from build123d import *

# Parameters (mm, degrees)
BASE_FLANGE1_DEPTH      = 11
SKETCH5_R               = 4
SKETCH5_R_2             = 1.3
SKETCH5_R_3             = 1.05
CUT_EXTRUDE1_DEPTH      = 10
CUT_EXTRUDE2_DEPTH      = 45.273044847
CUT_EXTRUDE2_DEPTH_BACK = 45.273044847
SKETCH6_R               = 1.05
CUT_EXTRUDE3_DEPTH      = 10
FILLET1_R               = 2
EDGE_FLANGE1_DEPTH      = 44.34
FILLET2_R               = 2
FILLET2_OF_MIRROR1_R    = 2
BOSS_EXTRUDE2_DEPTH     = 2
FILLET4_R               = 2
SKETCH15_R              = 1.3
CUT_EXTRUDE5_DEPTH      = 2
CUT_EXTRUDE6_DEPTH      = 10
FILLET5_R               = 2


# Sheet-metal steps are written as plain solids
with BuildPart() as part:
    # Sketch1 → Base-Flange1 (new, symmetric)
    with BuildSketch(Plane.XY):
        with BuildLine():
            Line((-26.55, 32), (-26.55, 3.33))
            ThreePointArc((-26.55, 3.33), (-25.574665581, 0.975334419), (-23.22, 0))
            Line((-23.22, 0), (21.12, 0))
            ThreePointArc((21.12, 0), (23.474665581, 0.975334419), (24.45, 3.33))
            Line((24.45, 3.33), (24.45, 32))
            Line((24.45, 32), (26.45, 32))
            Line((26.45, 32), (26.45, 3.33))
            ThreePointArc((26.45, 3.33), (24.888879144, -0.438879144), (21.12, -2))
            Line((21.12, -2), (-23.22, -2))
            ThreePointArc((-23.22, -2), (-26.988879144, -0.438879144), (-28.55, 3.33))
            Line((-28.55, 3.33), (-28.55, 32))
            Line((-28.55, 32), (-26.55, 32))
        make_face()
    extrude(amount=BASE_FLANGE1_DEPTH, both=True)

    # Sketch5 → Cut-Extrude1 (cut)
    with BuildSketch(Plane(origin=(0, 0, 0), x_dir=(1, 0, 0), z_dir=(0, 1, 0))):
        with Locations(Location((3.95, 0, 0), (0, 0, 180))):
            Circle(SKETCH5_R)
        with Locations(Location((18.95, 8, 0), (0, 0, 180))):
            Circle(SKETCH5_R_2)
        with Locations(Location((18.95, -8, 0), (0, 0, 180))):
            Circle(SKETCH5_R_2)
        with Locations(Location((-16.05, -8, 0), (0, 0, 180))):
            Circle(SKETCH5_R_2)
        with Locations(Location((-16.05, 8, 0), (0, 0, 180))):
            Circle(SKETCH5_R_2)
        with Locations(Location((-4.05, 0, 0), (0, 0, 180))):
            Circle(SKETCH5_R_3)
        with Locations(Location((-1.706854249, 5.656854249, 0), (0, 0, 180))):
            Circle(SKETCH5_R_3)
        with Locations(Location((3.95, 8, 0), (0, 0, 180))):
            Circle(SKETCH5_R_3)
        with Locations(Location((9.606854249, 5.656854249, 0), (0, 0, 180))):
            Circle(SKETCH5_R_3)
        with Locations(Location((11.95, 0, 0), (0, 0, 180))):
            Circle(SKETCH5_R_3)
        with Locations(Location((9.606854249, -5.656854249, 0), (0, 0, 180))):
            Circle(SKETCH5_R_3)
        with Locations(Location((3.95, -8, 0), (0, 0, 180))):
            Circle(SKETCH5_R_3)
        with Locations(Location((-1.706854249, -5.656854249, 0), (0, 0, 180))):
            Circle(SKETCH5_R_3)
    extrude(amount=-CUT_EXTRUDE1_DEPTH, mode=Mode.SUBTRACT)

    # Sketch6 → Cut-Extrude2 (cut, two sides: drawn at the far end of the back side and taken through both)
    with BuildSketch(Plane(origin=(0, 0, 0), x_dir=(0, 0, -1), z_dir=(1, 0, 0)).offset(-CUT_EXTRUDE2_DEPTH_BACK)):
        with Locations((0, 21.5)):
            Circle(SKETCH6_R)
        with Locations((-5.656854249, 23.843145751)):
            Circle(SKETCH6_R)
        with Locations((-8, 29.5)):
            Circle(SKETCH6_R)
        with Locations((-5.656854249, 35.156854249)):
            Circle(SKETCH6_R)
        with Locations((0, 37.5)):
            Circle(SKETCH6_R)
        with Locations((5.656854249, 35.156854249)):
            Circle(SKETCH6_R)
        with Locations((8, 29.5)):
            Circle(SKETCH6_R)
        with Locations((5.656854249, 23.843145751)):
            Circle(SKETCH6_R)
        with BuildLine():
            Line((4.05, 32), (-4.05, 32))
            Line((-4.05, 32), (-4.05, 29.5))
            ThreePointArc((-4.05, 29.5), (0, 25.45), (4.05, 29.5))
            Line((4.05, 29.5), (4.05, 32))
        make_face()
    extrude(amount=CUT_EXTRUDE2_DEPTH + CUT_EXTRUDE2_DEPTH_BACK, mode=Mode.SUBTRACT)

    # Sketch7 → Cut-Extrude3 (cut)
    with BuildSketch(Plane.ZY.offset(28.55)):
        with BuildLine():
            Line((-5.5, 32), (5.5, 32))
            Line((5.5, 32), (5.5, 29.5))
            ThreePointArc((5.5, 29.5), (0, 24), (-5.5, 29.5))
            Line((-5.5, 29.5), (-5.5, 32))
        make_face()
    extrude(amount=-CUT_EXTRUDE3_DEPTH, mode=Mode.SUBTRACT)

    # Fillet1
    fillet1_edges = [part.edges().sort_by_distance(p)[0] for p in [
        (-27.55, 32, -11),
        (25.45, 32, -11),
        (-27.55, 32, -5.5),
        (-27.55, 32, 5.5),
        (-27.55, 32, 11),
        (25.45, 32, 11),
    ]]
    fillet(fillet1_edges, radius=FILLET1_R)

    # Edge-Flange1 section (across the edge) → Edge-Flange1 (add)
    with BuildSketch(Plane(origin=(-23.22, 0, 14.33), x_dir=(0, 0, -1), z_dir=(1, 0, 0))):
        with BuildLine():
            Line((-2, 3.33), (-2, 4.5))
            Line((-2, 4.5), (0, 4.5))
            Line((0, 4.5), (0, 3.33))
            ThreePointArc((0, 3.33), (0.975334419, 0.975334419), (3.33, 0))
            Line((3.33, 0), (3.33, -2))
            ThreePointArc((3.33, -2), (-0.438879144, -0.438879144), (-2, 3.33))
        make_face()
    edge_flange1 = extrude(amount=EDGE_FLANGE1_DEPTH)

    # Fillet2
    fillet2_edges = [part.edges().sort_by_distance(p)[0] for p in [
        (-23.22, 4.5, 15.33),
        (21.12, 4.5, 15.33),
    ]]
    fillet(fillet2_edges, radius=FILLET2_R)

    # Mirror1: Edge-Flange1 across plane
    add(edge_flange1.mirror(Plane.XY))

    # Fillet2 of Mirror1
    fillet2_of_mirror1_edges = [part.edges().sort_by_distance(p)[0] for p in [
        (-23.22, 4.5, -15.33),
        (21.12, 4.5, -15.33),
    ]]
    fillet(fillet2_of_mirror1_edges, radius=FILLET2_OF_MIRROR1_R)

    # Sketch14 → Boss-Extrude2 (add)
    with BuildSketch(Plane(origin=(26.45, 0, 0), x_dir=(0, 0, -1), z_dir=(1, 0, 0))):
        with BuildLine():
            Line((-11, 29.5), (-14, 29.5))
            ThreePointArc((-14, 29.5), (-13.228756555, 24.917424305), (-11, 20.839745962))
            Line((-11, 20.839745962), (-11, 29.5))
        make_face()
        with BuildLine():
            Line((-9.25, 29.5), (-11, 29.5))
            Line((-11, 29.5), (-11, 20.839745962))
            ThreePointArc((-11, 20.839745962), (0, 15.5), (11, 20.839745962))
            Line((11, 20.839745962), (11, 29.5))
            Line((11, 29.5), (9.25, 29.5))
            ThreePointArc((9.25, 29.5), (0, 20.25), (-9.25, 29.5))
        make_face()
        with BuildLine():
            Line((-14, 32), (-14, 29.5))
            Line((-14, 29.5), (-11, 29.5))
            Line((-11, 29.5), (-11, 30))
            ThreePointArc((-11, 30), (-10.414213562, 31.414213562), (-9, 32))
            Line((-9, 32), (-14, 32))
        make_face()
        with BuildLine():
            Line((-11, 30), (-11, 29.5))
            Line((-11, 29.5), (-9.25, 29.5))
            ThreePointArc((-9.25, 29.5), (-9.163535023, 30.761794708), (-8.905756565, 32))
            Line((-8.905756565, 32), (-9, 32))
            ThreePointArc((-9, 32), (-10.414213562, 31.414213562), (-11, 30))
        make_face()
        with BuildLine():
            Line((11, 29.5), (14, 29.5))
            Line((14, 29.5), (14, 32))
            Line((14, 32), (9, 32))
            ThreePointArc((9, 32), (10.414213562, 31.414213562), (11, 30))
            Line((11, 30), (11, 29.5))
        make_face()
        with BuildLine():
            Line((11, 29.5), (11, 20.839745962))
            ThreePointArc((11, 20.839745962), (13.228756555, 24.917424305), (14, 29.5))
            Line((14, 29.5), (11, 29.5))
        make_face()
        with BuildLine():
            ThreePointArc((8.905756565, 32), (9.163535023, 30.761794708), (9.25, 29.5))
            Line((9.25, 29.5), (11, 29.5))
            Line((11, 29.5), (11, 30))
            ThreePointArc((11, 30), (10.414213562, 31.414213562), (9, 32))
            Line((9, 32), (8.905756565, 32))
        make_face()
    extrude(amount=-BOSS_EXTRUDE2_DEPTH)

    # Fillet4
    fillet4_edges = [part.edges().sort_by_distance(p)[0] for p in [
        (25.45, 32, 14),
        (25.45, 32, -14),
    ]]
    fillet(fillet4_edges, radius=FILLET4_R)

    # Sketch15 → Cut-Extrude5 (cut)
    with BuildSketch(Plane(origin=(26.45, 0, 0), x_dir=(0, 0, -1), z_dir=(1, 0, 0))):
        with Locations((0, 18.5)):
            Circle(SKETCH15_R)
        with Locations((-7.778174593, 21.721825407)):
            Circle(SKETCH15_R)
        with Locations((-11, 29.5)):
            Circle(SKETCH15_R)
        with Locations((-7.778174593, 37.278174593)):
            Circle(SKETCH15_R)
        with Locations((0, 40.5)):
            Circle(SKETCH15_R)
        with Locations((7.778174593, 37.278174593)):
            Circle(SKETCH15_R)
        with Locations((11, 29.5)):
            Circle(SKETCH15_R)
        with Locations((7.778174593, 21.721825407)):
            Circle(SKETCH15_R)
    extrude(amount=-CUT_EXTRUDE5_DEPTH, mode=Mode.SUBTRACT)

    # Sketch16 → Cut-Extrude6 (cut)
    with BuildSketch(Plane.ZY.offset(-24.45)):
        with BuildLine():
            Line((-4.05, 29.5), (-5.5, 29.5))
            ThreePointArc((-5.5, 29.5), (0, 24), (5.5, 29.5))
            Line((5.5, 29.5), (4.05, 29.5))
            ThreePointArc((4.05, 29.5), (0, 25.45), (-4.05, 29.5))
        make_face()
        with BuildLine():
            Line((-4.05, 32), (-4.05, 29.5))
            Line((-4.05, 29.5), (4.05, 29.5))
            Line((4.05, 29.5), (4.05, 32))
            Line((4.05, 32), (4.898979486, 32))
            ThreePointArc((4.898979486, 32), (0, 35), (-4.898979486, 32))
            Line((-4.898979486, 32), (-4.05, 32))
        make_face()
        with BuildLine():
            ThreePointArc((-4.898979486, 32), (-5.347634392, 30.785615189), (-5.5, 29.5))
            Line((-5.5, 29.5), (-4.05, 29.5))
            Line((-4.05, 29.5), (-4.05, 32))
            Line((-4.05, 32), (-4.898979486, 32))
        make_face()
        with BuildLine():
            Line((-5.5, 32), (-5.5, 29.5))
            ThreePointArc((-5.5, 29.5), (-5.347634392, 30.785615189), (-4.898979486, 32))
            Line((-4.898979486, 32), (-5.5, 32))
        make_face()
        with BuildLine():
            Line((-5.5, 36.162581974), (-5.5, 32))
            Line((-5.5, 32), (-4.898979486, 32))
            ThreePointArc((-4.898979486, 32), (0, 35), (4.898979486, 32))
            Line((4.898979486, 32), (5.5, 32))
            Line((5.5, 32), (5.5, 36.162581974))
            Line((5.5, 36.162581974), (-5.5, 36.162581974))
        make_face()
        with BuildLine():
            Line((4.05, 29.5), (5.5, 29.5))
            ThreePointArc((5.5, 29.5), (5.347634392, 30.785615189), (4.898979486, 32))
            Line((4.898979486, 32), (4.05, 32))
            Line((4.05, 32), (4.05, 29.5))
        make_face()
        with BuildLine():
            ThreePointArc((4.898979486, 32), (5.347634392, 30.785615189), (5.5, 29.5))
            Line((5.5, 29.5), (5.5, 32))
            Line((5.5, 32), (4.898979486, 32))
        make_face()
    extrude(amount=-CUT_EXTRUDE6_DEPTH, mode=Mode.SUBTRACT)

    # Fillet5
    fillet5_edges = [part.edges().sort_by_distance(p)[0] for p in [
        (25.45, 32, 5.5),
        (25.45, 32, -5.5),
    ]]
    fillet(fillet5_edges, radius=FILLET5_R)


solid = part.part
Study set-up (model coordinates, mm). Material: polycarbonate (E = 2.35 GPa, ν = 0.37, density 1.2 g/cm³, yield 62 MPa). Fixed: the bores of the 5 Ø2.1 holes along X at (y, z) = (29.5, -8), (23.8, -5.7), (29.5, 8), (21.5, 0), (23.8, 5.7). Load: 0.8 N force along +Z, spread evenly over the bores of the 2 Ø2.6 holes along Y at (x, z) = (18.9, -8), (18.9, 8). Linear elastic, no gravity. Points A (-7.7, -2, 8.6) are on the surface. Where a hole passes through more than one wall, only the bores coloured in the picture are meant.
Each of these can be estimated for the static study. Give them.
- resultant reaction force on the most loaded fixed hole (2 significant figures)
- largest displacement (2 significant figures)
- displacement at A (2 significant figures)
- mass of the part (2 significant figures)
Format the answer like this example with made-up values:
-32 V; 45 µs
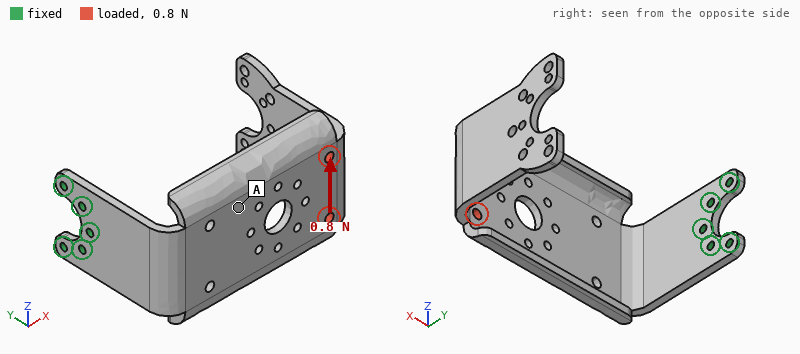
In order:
2.7 N; 0.80 mm; 0.27 mm; 7.1 g
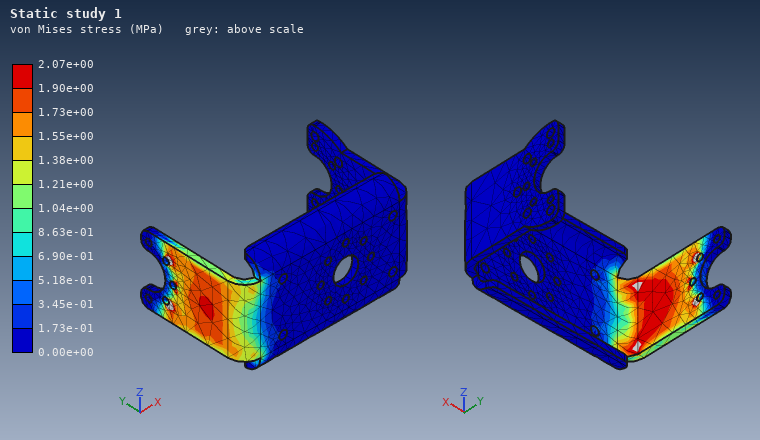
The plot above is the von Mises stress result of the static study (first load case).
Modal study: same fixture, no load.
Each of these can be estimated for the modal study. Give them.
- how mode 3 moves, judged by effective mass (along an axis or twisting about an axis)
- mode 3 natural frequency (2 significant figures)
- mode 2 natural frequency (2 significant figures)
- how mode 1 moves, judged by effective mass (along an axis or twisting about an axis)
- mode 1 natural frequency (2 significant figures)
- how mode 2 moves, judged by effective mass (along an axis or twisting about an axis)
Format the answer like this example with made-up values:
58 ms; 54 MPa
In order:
along X; 250 Hz; 87 Hz; along Y; 62 Hz; along Z
